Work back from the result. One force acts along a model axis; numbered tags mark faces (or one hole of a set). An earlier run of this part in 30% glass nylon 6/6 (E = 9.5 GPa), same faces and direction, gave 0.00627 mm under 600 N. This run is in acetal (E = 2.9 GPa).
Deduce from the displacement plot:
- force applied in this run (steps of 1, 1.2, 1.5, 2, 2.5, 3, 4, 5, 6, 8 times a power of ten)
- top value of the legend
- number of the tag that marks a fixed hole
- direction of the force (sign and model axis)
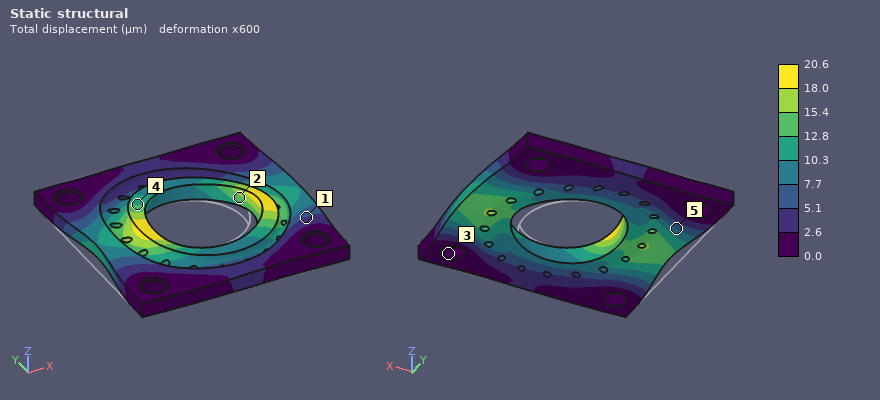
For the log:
600 N
20.6 µm
3
+X
